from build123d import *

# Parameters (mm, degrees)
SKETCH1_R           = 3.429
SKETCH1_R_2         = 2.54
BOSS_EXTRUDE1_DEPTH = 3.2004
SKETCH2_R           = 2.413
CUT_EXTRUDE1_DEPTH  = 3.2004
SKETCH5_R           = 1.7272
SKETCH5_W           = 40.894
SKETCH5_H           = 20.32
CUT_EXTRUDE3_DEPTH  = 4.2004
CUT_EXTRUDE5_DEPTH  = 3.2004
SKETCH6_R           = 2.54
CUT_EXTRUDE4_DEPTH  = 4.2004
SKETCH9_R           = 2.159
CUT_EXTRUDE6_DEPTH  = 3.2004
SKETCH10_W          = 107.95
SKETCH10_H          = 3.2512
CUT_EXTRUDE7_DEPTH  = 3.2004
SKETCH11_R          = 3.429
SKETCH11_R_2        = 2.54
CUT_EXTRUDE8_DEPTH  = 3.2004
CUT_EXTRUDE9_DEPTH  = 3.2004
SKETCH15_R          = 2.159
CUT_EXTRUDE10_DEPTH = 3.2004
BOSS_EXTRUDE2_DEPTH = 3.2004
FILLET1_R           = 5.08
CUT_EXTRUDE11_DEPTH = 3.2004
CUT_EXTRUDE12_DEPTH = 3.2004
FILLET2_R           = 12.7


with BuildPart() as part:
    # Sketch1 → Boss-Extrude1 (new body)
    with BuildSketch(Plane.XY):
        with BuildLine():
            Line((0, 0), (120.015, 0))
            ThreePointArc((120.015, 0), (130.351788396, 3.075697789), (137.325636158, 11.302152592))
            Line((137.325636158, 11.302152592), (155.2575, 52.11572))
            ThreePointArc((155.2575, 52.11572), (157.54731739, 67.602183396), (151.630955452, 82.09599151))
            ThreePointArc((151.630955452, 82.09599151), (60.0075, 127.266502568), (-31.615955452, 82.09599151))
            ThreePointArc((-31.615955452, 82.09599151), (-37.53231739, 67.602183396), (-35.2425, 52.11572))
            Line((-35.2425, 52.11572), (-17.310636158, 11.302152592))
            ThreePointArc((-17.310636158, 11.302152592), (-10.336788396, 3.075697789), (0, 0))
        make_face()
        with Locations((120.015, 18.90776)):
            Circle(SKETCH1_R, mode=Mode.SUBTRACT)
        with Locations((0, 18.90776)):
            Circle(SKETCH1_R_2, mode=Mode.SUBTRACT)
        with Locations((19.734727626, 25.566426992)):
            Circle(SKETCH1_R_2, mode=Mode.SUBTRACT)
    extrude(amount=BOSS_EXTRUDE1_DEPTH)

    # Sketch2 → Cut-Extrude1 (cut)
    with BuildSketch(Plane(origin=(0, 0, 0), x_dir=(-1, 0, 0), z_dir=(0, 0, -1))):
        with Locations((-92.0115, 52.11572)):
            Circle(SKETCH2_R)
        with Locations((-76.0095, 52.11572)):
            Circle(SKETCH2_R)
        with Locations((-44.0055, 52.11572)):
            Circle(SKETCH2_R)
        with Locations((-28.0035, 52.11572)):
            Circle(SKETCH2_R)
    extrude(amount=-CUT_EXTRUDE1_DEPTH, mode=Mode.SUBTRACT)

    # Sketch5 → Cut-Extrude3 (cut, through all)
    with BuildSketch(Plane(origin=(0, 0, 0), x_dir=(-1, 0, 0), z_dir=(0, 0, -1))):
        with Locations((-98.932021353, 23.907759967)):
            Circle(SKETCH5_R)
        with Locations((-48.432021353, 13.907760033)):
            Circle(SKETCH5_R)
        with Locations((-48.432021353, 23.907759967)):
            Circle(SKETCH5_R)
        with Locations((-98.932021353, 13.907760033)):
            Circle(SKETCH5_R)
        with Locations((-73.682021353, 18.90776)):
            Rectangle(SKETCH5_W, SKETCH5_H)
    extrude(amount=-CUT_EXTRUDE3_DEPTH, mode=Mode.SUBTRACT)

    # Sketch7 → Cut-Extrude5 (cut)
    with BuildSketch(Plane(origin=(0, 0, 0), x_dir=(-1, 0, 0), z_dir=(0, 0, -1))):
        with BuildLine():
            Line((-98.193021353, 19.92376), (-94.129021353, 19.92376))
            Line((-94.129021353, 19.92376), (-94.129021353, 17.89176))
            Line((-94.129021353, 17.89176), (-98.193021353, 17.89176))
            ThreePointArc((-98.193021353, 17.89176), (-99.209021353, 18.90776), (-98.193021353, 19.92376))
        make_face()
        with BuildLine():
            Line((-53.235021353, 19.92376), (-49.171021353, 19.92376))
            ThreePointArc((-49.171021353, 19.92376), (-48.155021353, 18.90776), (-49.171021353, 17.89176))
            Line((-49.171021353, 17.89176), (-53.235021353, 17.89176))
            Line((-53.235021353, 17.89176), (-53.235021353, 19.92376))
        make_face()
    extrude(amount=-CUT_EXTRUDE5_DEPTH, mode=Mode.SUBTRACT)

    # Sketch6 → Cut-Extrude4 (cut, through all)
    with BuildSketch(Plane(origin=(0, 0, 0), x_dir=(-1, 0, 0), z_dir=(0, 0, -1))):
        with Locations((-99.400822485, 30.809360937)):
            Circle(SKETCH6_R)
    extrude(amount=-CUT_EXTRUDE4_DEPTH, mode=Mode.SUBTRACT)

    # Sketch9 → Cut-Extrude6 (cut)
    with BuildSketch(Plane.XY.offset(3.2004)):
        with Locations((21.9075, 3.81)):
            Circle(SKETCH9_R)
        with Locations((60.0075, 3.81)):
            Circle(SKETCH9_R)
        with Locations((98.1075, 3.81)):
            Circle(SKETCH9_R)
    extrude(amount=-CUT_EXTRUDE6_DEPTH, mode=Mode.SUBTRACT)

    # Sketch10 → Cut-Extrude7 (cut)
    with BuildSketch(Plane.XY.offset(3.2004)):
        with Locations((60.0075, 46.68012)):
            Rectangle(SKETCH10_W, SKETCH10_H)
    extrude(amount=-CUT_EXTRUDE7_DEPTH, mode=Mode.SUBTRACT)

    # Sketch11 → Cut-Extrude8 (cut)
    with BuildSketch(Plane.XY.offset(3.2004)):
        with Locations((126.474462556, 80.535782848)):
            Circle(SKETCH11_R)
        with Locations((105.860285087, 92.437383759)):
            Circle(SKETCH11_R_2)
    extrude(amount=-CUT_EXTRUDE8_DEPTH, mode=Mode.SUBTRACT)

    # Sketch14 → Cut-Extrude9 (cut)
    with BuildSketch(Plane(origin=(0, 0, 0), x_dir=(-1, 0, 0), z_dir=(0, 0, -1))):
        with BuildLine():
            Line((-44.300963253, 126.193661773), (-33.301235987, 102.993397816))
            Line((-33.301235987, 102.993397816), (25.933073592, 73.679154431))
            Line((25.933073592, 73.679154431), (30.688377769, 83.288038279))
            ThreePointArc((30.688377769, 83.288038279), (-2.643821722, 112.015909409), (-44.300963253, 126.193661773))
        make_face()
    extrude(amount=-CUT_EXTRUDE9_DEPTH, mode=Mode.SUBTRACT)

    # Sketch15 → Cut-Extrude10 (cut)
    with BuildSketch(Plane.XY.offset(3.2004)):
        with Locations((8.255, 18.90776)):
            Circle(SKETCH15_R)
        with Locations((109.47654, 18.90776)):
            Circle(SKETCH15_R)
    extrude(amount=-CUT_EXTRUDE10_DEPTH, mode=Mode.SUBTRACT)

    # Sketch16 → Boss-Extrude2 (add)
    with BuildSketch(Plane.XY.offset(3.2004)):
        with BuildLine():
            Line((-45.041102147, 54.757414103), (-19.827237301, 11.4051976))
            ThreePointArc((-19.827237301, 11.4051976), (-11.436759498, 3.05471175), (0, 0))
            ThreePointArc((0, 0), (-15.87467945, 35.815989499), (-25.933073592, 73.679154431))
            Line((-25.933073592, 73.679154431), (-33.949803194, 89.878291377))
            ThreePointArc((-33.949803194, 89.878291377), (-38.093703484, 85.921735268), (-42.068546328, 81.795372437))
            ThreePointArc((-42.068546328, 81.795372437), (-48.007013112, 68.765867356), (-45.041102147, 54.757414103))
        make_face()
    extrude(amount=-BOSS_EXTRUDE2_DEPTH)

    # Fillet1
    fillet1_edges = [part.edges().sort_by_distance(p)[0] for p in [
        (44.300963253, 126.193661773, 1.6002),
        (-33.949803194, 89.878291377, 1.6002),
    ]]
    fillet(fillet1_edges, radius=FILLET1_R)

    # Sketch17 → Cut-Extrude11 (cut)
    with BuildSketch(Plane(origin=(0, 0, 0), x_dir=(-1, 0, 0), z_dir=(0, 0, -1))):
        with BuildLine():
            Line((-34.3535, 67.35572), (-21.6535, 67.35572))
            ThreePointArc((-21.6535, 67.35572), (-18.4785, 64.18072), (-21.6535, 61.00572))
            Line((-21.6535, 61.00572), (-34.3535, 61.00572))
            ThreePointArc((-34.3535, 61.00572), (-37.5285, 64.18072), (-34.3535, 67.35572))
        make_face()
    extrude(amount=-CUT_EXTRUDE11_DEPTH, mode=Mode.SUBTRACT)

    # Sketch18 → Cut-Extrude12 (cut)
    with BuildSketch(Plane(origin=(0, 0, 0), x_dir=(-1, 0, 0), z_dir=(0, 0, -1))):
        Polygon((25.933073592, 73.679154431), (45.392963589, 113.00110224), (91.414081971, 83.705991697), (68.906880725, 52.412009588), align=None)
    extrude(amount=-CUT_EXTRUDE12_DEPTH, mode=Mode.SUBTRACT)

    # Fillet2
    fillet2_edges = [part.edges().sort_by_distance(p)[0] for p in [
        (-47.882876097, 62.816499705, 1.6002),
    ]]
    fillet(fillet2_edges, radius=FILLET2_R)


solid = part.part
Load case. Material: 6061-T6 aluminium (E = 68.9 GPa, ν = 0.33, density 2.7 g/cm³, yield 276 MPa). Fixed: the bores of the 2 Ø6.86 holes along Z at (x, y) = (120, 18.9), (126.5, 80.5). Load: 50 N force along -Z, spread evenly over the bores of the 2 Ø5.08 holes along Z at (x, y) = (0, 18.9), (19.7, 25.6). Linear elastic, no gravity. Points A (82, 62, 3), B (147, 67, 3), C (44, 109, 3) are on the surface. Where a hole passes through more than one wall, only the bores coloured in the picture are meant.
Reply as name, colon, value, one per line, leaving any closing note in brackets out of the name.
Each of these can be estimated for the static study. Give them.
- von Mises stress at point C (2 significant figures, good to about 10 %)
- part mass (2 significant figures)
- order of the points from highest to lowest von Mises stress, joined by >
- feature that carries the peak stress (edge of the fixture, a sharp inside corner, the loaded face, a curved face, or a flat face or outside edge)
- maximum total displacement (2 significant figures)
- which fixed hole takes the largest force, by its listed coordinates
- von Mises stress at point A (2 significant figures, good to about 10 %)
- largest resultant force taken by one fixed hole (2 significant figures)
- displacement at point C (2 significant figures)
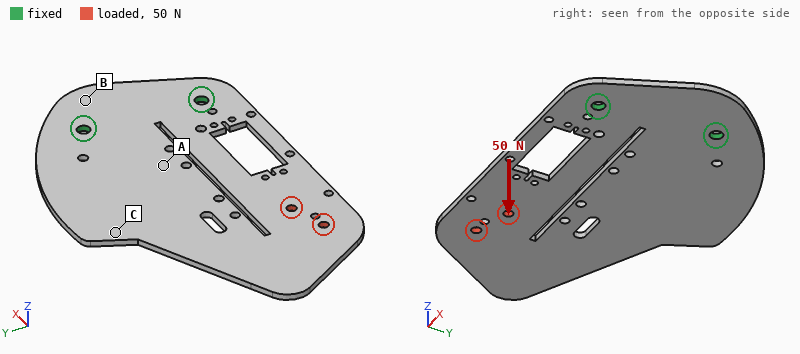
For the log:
von Mises stress at point C: 11 MPa
part mass: 150 g
order of the points from highest to lowest von Mises stress, joined by >: A > C > B
feature that carries the peak stress: a curved face
maximum total displacement: 2.5 mm
which fixed hole takes the largest force, by its listed coordinates: (120, 18.9)
von Mises stress at point A: 20 MPa
largest resultant force taken by one fixed hole: 42 N
displacement at point C: 0.61 mm
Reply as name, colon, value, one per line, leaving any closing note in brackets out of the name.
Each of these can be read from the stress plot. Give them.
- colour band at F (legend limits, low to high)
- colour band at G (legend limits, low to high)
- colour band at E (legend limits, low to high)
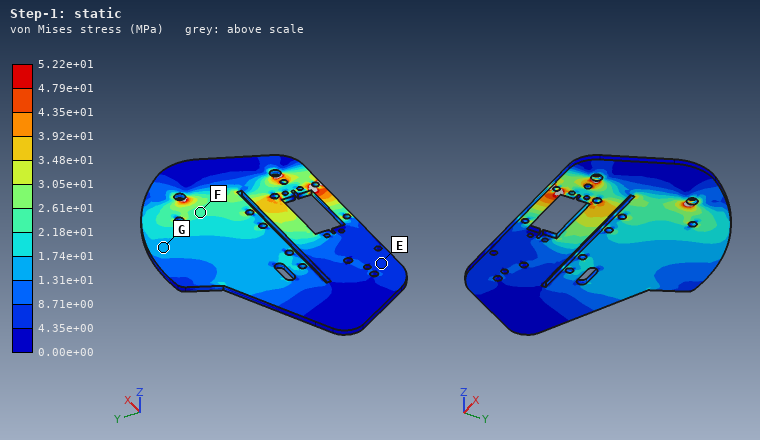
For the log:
colour band at F: 2.18e+01 to 2.61e+01 MPa
colour band at G: 1.31e+01 to 1.74e+01 MPa
colour band at E: 4.35e+00 to 8.71e+00 MPa
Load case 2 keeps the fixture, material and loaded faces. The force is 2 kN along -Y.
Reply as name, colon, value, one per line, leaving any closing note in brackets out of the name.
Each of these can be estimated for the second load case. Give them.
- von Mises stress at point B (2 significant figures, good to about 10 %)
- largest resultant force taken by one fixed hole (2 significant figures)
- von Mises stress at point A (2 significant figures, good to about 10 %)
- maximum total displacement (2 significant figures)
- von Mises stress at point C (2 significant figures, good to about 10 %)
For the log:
von Mises stress at point B: 18 MPa
largest resultant force taken by one fixed hole: 3.6 kN
von Mises stress at point A: 16 MPa
maximum total displacement: 0.30 mm
von Mises stress at point C: 12 MPa
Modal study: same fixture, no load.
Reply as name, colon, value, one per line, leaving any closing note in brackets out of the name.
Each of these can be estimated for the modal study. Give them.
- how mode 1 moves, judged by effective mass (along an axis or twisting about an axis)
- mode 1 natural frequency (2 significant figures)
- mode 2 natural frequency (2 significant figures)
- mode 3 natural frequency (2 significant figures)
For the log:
how mode 1 moves, judged by effective mass: along Z
mode 1 natural frequency: 110 Hz
mode 2 natural frequency: 370 Hz
mode 3 natural frequency: 630 Hz
